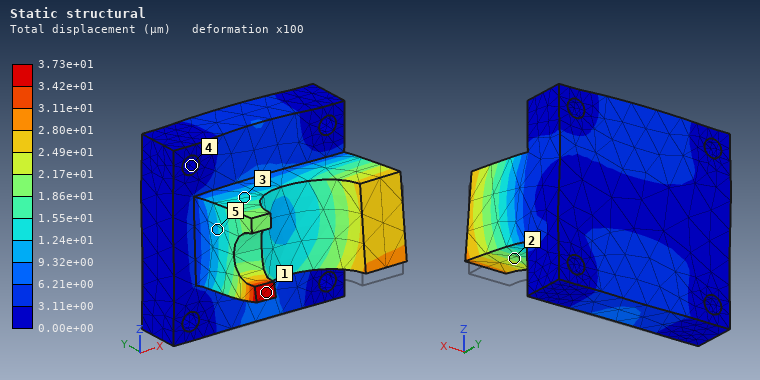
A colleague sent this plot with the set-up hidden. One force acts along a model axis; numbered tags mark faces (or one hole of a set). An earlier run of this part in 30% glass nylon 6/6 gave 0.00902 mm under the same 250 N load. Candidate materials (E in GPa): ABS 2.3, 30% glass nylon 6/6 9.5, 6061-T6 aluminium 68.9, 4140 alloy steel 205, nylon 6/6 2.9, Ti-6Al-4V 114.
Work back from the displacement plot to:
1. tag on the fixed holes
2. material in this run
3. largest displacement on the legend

4
ABS
3.73e+01 µm
